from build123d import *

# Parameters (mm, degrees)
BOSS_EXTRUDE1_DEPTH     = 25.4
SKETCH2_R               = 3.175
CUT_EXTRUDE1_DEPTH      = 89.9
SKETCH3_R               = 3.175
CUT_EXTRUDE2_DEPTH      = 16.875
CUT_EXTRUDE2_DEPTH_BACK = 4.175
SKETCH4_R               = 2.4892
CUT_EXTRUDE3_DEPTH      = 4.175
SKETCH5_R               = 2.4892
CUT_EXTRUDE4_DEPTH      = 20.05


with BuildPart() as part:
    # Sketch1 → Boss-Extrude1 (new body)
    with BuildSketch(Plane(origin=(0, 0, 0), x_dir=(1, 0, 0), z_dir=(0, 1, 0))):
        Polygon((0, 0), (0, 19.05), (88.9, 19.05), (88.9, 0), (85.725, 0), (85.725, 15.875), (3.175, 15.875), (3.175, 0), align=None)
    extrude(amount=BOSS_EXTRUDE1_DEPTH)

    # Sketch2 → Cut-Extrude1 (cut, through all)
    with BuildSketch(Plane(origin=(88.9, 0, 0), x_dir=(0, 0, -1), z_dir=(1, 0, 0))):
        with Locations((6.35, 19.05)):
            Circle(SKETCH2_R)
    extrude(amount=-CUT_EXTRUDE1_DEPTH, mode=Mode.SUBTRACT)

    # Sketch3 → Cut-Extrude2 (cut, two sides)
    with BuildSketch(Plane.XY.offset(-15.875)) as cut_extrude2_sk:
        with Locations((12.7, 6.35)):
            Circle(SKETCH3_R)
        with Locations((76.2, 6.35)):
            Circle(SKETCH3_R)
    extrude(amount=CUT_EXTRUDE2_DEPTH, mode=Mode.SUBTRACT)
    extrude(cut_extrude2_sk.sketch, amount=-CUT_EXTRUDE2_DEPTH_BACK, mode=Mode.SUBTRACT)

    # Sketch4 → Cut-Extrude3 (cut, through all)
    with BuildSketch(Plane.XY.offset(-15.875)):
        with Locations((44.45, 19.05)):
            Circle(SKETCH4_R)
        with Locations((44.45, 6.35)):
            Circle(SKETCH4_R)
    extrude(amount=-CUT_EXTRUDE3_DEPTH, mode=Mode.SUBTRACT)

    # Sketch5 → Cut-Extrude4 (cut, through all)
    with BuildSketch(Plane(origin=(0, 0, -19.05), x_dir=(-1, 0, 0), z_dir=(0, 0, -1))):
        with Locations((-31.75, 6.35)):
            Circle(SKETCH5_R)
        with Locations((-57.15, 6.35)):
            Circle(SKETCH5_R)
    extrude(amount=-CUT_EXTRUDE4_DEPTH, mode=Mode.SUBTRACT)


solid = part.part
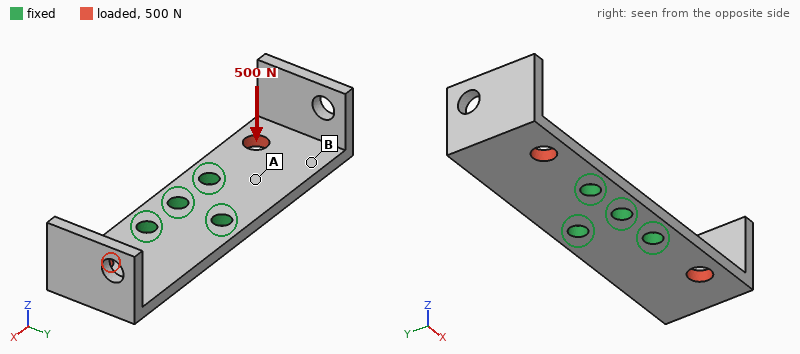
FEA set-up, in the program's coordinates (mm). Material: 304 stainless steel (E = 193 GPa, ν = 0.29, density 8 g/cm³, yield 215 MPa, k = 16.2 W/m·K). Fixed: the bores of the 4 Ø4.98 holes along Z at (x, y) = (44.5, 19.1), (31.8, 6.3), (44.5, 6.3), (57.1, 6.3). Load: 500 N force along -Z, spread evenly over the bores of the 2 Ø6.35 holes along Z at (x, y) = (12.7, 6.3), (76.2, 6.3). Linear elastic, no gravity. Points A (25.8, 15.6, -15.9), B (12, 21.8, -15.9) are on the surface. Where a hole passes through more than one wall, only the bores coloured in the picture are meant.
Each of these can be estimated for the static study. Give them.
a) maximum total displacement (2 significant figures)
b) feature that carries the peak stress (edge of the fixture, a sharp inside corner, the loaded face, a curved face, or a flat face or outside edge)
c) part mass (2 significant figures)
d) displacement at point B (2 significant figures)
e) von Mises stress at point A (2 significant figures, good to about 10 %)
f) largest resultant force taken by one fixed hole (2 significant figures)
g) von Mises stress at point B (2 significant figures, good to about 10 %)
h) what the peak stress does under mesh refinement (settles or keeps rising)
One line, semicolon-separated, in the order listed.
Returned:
0.11 mm; edge of the fixture; 73 g; 0.041 mm; 59 MPa; 360 N; 18 MPa; keeps rising
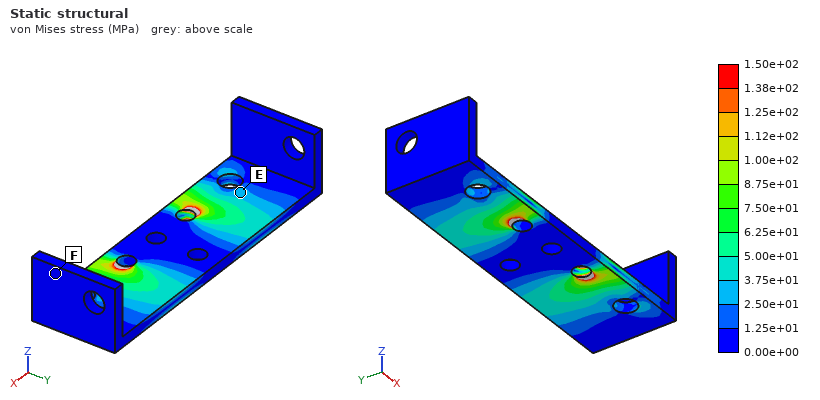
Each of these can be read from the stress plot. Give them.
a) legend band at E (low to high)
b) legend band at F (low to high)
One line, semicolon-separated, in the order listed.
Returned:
2.50e+01 to 3.75e+01 MPa; 0.00e+00 to 1.25e+01 MPa
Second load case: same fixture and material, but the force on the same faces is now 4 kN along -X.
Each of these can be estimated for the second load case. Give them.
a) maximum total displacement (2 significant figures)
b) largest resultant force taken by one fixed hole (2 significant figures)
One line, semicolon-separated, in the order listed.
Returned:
10.0 µm; 1.7 kN
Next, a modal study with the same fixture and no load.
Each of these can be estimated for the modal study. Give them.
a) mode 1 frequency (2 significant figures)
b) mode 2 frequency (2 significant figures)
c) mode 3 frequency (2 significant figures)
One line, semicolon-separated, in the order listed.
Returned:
1400 Hz; 1400 Hz; 2900 Hz
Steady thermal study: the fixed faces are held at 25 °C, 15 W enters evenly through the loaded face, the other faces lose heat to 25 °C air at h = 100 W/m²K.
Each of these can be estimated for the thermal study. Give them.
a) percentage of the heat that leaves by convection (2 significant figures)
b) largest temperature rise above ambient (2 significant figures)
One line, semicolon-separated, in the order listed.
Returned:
73 %; 64 K
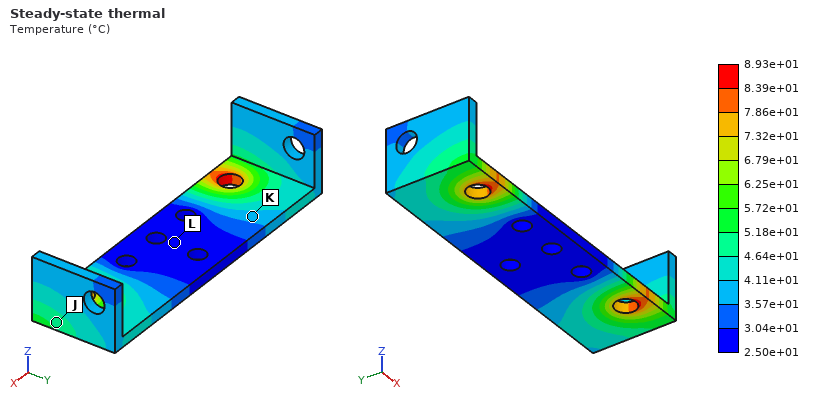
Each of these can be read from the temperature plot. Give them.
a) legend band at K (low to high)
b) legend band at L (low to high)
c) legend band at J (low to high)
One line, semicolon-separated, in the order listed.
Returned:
3.57e+01 to 4.11e+01 °C; 2.50e+01 to 3.04e+01 °C; 4.64e+01 to 5.18e+01 °C
